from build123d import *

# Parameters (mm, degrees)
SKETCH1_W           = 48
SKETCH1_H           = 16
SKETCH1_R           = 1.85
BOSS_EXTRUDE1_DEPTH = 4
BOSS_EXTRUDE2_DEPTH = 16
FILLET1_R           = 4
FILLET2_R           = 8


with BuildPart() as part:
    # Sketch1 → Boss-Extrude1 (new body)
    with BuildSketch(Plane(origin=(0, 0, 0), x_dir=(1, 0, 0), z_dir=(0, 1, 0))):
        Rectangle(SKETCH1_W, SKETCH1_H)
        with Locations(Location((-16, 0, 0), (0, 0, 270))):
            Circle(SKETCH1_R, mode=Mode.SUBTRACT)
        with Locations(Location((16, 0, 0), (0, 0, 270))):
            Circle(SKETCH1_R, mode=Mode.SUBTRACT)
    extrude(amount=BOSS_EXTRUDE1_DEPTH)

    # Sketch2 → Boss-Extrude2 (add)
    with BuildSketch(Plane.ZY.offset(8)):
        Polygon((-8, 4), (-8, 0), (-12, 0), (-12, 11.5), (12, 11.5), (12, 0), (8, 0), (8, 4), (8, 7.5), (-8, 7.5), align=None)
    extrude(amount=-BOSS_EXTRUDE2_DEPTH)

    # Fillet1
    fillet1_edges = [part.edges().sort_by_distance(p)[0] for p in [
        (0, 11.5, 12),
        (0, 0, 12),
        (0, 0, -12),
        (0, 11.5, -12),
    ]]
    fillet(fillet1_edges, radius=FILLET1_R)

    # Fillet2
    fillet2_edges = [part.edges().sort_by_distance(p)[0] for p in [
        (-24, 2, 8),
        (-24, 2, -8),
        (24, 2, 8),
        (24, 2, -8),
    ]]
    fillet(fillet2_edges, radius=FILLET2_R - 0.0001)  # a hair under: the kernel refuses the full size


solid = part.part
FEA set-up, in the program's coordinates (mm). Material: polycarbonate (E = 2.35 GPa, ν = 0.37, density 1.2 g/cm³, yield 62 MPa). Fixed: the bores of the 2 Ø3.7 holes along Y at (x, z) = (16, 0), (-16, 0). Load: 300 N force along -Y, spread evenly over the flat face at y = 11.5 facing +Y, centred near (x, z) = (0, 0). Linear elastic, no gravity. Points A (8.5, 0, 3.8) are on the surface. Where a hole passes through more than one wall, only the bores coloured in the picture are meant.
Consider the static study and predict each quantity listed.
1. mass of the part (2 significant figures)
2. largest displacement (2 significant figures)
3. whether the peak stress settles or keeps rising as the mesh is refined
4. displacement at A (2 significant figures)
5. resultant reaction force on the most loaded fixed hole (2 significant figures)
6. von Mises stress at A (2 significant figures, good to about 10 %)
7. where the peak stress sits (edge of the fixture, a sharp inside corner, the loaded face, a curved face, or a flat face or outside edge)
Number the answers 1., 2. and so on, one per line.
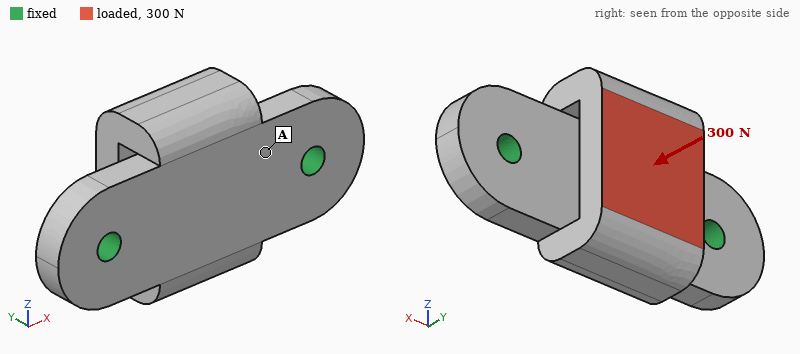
1. 6.1 g
2. 0.28 mm
3. keeps rising
4. 0.11 mm
5. 150 N
6. 6.9 MPa
7. edge of the fixture
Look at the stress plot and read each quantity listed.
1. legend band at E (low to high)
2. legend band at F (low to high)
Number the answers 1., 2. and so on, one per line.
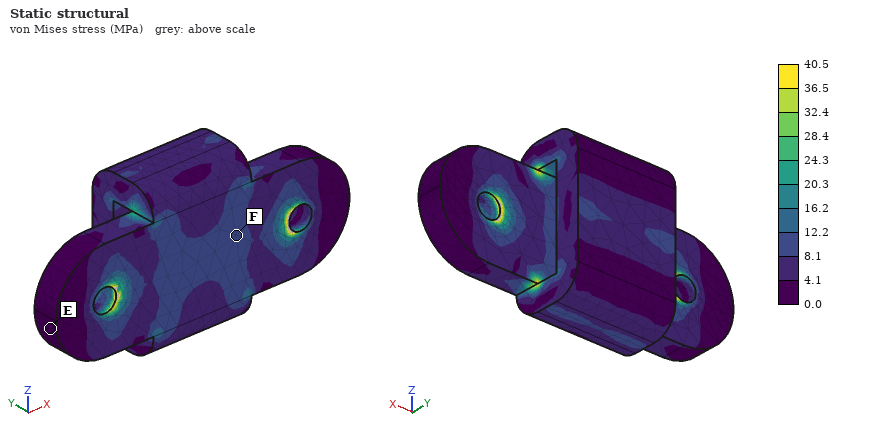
1. 0.0 to 4.1 MPa
2. 8.1 to 12.2 MPa
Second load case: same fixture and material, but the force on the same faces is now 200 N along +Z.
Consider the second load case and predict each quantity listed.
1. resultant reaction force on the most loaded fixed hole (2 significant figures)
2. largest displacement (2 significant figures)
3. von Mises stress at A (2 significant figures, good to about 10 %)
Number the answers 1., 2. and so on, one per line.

1. 100 N
2. 0.52 mm
3. 12 MPa
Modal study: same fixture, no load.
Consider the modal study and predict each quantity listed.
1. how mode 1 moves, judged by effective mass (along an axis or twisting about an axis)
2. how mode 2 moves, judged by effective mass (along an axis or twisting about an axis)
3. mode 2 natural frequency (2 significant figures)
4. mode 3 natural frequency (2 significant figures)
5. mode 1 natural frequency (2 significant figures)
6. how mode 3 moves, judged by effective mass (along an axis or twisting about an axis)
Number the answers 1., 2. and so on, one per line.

1. along Z
2. along Y
3. 3200 Hz
4. 4500 Hz
5. 2100 Hz
6. along X
